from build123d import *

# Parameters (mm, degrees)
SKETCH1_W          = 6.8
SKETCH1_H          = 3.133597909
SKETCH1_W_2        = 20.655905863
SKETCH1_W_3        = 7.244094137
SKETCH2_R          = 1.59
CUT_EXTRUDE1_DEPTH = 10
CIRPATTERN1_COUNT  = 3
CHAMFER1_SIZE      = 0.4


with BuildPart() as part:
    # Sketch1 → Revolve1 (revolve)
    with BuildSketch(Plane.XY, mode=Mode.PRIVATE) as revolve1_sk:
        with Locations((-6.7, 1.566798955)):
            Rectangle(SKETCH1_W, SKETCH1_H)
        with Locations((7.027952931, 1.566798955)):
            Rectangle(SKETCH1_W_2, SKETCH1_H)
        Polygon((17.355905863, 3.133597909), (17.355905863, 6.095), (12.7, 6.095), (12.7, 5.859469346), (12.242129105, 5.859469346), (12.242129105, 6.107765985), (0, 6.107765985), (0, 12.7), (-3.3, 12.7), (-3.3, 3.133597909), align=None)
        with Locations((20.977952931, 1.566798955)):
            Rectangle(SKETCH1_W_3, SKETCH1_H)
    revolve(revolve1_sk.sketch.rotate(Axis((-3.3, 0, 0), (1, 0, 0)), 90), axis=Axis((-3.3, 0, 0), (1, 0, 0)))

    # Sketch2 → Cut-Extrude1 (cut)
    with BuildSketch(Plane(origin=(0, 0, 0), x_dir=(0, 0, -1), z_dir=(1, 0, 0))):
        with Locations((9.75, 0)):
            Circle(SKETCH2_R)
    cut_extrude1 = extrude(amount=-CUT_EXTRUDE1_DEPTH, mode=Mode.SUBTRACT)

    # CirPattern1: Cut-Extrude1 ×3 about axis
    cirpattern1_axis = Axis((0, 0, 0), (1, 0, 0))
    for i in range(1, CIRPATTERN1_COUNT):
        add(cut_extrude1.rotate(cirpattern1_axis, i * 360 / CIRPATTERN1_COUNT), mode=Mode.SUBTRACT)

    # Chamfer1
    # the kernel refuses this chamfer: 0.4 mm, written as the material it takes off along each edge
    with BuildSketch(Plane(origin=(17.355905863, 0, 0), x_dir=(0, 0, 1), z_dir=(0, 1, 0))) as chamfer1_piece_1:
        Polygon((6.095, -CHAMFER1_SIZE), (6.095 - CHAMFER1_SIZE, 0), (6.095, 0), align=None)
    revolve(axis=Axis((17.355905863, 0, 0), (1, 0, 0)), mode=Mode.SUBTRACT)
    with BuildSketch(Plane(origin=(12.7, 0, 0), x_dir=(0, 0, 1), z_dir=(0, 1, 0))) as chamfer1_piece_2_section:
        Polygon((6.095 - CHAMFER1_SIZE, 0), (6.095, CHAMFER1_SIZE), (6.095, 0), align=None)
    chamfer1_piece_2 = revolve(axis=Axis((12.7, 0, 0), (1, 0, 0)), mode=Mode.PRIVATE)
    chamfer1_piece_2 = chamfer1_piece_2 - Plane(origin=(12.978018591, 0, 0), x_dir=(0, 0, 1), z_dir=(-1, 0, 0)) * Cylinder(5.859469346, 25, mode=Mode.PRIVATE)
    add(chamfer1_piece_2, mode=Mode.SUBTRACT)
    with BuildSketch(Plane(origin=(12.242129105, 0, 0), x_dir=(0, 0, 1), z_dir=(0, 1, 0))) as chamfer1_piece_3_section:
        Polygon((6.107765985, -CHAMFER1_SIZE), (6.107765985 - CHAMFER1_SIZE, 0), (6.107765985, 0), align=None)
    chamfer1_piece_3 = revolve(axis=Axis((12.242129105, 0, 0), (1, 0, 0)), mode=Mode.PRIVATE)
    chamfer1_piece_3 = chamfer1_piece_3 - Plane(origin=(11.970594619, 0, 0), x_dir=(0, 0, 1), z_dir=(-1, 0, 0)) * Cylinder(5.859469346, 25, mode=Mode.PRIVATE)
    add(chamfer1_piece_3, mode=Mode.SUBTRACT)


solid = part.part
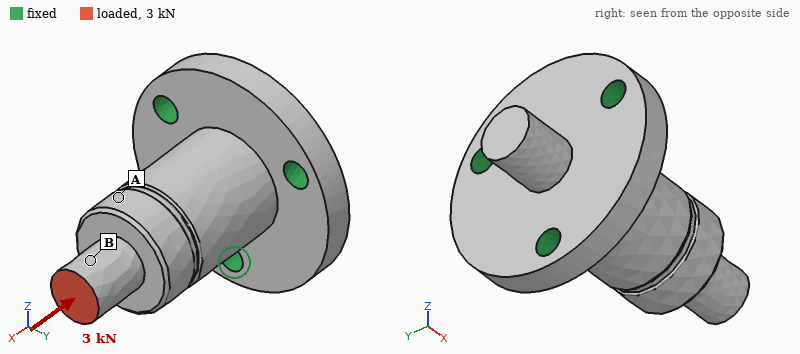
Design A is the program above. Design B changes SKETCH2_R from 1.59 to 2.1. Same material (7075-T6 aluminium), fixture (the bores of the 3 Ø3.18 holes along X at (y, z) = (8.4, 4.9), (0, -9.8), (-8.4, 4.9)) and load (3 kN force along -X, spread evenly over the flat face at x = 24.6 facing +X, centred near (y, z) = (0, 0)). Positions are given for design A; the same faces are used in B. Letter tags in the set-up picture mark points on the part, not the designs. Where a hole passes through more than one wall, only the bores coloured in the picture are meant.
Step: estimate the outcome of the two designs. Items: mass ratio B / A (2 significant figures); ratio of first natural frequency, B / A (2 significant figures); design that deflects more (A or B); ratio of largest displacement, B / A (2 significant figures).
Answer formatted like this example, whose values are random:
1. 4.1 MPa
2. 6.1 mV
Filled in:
1. 0.99
2. 1.1
3. A
4. 0.92
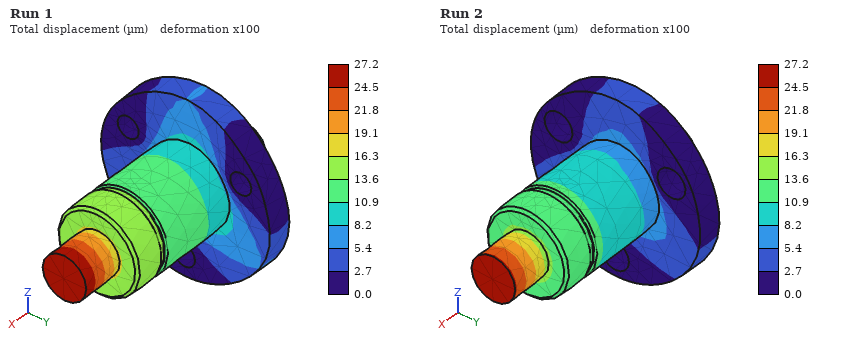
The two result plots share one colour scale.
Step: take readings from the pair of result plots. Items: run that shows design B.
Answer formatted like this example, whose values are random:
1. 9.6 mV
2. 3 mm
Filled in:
1. Run 2
